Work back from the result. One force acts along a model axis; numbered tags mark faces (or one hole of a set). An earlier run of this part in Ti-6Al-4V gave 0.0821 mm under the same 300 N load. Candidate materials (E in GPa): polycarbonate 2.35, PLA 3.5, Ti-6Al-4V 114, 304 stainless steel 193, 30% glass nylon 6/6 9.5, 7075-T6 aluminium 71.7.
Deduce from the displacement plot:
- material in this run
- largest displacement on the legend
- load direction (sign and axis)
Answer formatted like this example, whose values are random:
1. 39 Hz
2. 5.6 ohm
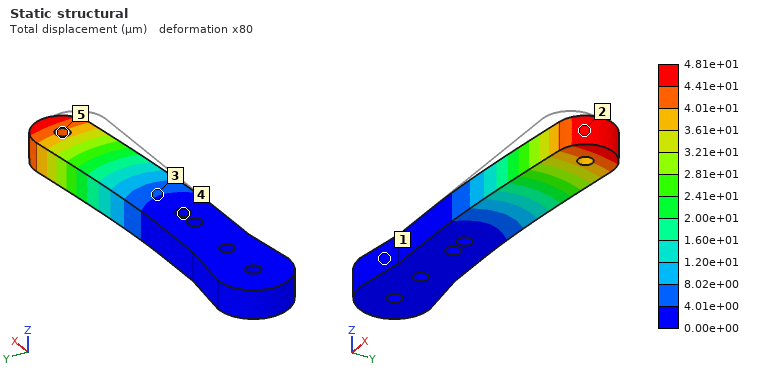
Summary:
1. 304 stainless steel
2. 4.81e+01 µm
3. +Y
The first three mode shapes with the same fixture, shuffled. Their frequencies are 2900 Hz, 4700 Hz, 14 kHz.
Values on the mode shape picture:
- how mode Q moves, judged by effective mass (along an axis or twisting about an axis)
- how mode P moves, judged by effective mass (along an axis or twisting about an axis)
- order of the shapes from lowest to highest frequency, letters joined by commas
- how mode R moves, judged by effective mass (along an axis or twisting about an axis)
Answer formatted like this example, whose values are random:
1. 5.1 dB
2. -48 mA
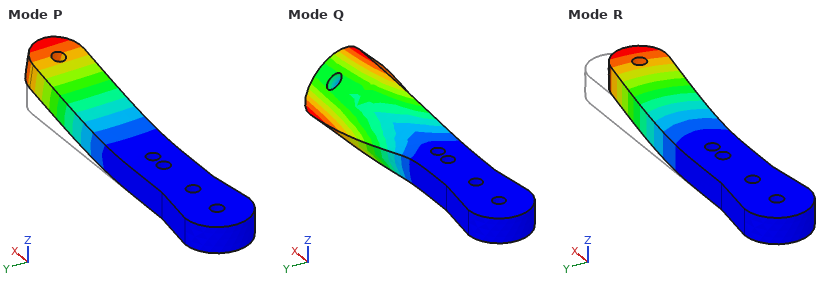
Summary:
1. twisting about X
2. along Z
3. P, R, Q
4. along Y
